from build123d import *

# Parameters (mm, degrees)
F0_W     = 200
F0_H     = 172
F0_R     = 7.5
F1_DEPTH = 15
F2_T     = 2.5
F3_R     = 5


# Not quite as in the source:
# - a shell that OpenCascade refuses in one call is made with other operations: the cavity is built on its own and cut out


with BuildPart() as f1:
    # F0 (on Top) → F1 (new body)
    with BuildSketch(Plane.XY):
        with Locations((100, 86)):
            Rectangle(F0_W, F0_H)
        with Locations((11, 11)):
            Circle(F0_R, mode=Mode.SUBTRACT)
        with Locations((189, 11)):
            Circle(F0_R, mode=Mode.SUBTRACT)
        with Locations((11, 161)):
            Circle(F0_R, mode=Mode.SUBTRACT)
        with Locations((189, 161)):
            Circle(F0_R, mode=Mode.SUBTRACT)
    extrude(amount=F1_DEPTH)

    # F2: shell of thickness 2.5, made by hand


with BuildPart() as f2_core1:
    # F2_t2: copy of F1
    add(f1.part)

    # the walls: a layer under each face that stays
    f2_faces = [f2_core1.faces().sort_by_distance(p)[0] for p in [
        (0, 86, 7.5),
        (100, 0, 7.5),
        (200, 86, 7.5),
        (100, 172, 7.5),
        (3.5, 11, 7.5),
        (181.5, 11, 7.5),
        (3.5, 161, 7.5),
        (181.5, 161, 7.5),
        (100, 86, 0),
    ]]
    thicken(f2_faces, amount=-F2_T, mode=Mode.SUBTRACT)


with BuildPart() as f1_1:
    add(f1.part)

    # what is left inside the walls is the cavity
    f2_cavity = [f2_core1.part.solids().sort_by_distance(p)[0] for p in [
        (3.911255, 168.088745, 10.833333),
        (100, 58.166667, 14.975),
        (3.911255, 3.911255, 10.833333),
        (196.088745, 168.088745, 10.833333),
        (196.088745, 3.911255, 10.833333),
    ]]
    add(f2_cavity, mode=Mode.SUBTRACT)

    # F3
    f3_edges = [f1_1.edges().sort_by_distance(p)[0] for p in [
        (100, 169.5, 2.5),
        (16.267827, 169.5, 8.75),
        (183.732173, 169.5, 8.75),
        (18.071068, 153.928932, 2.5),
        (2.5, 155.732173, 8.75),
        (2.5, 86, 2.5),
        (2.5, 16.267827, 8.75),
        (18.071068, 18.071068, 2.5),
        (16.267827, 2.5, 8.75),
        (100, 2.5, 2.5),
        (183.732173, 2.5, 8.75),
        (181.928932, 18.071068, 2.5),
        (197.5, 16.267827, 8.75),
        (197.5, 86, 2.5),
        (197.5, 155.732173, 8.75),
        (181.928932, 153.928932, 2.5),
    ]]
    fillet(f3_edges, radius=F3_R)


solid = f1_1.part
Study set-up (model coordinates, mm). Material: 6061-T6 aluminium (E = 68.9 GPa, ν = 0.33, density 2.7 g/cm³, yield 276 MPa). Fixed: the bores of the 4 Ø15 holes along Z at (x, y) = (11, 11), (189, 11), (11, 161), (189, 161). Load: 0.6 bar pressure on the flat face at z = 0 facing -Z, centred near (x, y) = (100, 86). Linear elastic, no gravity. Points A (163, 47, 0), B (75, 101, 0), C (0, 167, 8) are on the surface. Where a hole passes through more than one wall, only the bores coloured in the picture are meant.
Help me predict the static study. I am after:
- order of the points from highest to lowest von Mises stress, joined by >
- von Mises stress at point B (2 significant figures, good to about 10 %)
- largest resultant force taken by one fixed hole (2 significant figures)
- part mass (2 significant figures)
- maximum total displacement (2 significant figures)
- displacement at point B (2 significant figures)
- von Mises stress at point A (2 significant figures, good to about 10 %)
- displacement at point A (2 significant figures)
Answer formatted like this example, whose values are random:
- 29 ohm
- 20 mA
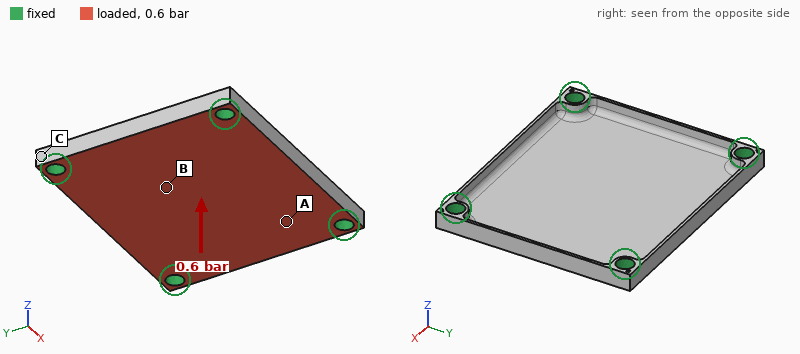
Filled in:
- B > A > C
- 55 MPa
- 650 N
- 320 g
- 1.4 mm
- 1.2 mm
- 24 MPa
- 0.44 mm
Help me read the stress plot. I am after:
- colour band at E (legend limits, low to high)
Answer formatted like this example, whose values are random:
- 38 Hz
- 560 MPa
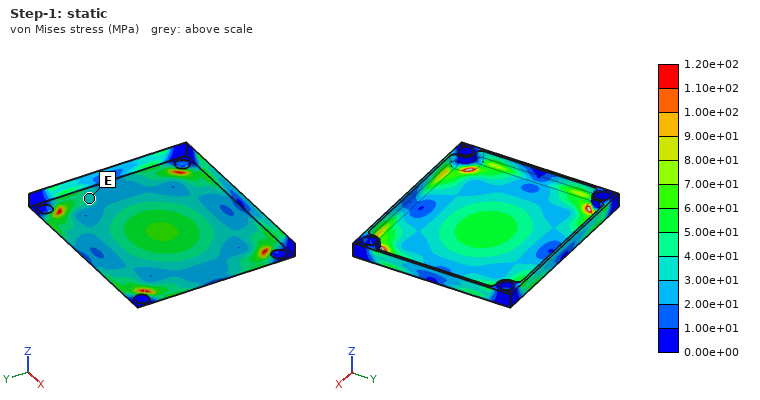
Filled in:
- 3.00e+01 to 4.00e+01 MPa
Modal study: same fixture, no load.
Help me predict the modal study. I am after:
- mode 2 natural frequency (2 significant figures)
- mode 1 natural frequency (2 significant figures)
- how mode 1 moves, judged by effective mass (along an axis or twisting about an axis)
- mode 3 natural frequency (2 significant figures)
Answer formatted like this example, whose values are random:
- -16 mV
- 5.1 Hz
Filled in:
- 1100 Hz
- 510 Hz
- along Z
- 1100 Hz
